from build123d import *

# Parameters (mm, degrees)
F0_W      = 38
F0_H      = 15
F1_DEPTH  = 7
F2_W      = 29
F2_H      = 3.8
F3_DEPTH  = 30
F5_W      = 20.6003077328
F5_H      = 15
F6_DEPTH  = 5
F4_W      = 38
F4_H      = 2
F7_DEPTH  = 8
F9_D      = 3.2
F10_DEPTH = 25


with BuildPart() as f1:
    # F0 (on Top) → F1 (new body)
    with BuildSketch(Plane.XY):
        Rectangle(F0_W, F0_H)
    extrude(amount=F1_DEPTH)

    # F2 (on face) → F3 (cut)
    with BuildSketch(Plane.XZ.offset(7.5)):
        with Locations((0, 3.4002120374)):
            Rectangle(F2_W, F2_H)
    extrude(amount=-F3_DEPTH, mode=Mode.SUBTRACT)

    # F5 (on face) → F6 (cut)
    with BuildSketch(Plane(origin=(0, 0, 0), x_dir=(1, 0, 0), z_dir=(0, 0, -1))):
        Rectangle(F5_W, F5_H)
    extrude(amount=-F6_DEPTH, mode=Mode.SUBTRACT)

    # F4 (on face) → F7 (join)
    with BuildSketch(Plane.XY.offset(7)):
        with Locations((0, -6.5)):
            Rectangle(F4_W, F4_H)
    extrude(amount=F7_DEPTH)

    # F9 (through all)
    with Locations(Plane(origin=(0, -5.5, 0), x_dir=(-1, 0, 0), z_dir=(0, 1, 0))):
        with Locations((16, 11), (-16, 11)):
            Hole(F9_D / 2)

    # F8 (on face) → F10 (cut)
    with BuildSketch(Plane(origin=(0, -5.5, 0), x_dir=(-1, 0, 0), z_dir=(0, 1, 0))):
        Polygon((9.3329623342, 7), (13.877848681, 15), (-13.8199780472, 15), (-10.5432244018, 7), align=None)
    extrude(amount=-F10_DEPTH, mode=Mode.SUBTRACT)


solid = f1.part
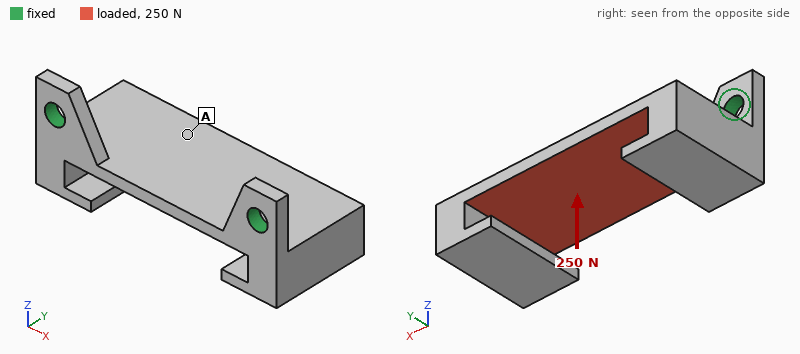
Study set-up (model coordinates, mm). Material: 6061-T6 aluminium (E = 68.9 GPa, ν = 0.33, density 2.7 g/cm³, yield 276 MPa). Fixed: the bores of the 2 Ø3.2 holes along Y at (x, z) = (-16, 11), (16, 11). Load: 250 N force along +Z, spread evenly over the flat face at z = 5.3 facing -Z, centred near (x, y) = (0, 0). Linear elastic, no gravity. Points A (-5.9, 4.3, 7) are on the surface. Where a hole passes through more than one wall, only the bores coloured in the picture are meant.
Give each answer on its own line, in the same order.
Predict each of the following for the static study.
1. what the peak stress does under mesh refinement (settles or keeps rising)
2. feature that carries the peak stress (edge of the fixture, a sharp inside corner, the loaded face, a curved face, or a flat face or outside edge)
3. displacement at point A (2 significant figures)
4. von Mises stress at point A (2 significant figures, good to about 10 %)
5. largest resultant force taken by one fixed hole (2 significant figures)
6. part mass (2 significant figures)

keeps rising
edge of the fixture
0.13 mm
26 MPa
150 N
5.6 g
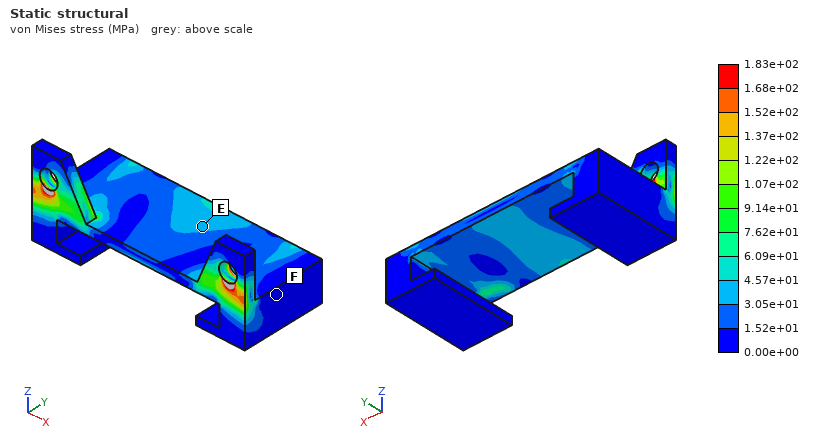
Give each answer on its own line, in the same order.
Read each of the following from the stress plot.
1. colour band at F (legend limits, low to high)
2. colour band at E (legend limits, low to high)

0.00e+00 to 1.52e+01 MPa
3.05e+01 to 4.57e+01 MPa
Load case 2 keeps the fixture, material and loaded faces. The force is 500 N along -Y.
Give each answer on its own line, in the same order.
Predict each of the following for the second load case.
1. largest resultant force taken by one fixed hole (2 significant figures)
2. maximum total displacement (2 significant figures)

270 N
0.13 mm
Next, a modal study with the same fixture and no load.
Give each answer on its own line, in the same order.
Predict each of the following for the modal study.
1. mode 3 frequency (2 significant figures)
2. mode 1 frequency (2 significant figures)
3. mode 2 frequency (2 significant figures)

10 kHz
3300 Hz
4700 Hz
